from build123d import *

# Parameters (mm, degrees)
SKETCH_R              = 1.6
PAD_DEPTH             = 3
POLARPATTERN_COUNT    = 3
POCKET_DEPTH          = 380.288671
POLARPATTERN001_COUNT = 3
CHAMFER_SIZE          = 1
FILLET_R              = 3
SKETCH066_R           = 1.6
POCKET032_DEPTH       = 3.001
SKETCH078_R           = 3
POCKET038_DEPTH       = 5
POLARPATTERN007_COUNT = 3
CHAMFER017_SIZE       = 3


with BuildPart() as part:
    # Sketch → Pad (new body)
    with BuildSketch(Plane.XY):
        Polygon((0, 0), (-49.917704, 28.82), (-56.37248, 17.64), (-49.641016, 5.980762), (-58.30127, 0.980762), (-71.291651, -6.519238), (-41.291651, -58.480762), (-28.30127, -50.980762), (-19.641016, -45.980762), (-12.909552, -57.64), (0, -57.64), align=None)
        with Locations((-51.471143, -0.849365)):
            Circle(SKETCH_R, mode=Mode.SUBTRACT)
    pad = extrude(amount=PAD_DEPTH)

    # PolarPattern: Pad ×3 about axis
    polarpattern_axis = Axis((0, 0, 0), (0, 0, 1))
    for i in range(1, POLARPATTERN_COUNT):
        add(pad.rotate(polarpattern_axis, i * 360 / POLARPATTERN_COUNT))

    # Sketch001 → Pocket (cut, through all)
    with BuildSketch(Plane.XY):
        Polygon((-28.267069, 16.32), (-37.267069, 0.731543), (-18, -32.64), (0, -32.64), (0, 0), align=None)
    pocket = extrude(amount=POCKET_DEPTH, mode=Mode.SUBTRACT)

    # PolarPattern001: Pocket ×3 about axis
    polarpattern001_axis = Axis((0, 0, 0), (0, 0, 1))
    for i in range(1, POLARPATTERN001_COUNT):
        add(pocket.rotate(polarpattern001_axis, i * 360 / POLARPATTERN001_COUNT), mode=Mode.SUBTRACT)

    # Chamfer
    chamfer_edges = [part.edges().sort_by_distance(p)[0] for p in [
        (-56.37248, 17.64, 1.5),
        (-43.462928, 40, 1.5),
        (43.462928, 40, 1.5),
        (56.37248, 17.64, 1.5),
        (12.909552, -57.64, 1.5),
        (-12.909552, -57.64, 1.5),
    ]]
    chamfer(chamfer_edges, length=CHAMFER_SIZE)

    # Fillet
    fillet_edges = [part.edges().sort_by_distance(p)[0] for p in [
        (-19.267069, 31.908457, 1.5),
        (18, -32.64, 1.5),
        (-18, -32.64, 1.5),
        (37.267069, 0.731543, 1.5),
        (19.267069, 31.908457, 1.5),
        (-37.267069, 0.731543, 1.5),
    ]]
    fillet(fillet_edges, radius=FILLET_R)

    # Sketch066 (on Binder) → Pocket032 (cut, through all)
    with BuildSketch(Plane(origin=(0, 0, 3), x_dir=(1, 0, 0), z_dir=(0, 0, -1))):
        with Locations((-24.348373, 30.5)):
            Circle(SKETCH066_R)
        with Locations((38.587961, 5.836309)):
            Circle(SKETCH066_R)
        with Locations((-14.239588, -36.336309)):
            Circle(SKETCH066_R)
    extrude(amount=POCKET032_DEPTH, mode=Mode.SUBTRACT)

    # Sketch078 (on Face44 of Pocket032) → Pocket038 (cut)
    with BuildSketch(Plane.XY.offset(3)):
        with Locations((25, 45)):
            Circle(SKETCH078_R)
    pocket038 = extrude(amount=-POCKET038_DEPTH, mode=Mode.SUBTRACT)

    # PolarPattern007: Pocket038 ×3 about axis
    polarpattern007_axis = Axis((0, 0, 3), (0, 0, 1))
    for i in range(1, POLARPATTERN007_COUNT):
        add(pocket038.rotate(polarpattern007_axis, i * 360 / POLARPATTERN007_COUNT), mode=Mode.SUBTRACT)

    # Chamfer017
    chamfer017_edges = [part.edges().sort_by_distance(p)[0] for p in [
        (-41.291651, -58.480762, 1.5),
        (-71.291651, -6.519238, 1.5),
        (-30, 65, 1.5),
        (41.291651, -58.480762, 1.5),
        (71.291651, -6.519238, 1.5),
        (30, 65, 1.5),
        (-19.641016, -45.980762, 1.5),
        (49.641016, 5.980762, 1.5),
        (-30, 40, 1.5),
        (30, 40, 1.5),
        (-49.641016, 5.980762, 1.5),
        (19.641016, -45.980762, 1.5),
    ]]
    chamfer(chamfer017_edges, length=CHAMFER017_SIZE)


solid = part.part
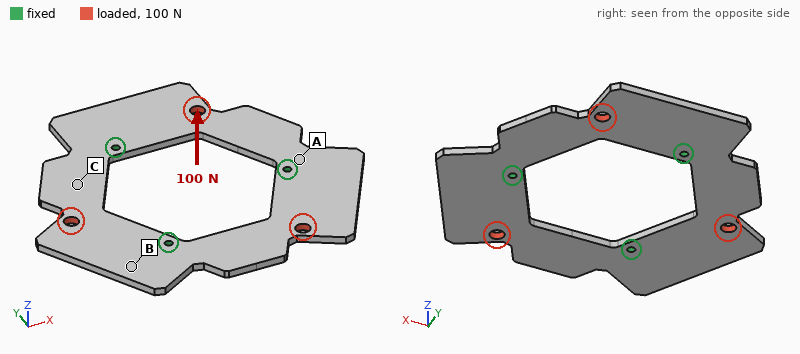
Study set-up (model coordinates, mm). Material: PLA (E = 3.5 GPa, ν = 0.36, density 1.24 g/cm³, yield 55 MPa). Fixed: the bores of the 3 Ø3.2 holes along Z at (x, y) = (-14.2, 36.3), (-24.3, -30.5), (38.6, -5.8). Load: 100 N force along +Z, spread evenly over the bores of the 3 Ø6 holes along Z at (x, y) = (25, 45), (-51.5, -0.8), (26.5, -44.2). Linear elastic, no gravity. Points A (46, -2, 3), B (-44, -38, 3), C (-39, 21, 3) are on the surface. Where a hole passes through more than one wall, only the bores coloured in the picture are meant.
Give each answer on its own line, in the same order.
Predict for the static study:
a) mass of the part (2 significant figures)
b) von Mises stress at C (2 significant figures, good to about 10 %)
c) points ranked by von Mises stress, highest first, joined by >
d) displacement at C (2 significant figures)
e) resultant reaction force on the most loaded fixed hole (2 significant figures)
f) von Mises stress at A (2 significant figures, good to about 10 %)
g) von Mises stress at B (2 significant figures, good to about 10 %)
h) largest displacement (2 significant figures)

31 g
4.3 MPa
A > B > C
0.69 mm
33 N
11 MPa
7.4 MPa
2.0 mm
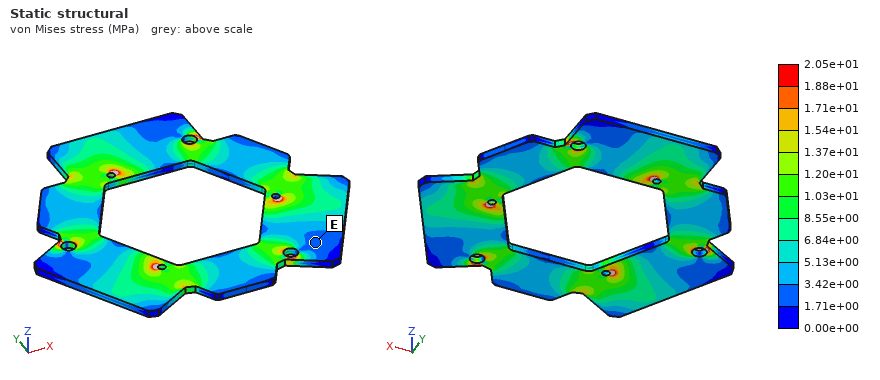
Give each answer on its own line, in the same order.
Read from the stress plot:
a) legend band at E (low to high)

1.71e+00 to 3.42e+00 MPa
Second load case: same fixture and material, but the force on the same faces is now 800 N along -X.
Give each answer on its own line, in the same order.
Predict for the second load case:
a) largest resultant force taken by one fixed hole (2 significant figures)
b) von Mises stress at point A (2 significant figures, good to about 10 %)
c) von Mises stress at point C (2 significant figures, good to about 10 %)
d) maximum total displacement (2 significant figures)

390 N
1.9 MPa
2.9 MPa
0.12 mm
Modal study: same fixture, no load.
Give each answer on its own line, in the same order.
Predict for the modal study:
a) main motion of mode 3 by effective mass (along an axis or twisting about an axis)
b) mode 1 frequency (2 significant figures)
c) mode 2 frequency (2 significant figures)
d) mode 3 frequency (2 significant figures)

along Z
350 Hz
350 Hz
420 Hz
